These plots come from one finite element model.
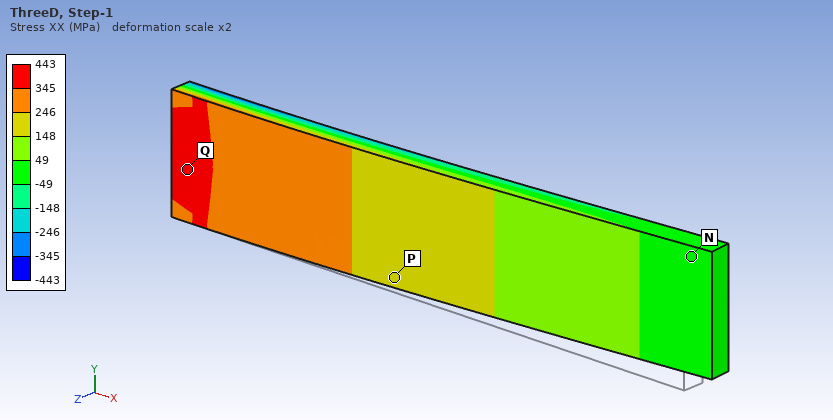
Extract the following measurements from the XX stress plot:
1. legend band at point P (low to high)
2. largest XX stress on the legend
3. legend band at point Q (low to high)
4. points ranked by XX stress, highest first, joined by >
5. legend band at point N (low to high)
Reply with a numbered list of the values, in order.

1. 148 to 246 MPa
2. 443 MPa
3. 345 to 443 MPa
4. Q > P > N
5. -49 to 49 MPa
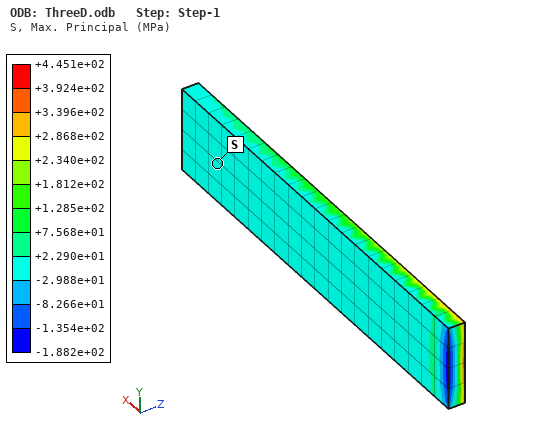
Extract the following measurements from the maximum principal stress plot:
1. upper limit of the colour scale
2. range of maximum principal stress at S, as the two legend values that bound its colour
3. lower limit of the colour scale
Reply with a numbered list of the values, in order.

1. +4.451e+02 MPa
2. -2.988e+01 to +2.290e+01 MPa
3. -1.882e+02 MPa
